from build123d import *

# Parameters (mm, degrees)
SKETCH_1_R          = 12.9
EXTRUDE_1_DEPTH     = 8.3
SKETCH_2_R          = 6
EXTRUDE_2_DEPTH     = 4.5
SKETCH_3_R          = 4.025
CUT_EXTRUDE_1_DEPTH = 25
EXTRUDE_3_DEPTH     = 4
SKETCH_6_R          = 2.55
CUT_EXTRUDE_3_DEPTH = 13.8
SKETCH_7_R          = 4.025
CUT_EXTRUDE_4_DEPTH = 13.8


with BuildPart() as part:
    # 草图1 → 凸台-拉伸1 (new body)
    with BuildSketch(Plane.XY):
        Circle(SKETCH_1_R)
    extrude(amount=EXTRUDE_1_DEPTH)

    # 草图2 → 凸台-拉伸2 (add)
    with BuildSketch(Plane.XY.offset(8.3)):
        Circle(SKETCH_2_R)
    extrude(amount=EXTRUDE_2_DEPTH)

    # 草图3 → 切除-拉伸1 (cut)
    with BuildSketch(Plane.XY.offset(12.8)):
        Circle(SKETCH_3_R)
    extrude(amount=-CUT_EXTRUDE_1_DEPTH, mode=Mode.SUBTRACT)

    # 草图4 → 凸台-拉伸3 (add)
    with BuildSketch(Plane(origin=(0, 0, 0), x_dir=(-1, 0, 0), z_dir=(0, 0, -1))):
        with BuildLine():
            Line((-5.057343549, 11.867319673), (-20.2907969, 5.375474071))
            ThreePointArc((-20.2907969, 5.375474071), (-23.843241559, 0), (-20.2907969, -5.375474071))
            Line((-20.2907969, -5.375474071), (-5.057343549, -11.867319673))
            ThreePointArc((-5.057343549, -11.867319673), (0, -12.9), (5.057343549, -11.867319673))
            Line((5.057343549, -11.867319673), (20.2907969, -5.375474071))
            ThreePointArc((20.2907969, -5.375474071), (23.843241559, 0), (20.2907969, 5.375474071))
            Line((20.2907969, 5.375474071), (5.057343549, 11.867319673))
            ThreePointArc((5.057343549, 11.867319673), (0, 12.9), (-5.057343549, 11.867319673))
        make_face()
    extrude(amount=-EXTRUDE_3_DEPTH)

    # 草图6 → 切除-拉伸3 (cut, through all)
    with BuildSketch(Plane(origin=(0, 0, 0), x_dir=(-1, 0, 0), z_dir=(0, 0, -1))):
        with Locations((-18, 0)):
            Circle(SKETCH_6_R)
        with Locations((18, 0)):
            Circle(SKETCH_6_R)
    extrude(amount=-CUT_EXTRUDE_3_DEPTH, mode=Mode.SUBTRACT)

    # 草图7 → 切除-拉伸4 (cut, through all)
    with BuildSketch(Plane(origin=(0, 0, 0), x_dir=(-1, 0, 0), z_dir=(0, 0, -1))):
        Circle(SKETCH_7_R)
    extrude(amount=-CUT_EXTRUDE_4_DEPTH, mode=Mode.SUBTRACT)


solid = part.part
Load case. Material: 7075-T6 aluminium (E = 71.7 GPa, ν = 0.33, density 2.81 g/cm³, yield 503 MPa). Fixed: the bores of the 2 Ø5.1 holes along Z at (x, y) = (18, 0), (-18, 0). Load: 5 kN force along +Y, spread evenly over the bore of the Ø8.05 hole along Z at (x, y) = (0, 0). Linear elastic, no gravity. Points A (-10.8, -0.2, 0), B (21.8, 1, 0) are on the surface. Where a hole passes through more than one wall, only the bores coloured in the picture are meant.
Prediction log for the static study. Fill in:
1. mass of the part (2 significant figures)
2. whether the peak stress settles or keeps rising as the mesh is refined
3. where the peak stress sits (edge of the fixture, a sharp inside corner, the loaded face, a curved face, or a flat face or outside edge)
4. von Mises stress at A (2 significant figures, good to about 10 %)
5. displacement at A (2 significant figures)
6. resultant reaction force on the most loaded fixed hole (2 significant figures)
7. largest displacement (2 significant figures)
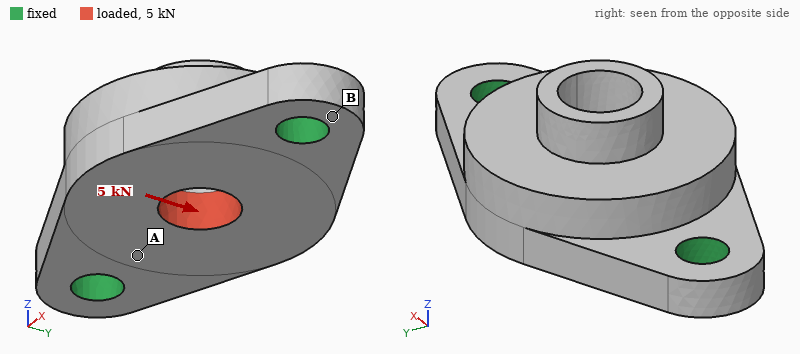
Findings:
15 g
keeps rising
edge of the fixture
49 MPa
12 µm
2.5 kN
23 µm
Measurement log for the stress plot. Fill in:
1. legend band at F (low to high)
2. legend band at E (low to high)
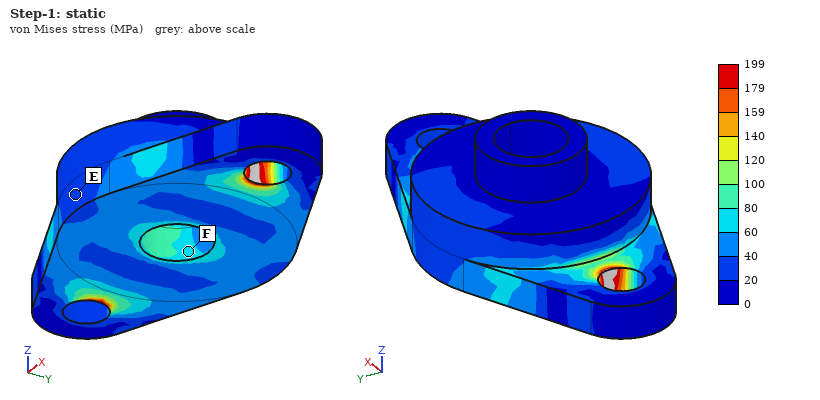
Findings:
60 to 80 MPa
20 to 40 MPa
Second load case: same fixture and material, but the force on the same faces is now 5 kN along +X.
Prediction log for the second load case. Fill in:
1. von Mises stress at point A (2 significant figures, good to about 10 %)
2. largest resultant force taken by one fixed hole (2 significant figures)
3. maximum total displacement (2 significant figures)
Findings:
62 MPa
2.5 kN
10 µm
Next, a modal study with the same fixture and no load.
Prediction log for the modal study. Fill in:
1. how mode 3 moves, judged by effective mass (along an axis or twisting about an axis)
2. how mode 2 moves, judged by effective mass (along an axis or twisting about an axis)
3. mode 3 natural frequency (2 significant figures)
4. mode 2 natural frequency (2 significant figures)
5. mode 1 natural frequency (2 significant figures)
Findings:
along Y
along Z
27 kHz
16 kHz
11 kHz
